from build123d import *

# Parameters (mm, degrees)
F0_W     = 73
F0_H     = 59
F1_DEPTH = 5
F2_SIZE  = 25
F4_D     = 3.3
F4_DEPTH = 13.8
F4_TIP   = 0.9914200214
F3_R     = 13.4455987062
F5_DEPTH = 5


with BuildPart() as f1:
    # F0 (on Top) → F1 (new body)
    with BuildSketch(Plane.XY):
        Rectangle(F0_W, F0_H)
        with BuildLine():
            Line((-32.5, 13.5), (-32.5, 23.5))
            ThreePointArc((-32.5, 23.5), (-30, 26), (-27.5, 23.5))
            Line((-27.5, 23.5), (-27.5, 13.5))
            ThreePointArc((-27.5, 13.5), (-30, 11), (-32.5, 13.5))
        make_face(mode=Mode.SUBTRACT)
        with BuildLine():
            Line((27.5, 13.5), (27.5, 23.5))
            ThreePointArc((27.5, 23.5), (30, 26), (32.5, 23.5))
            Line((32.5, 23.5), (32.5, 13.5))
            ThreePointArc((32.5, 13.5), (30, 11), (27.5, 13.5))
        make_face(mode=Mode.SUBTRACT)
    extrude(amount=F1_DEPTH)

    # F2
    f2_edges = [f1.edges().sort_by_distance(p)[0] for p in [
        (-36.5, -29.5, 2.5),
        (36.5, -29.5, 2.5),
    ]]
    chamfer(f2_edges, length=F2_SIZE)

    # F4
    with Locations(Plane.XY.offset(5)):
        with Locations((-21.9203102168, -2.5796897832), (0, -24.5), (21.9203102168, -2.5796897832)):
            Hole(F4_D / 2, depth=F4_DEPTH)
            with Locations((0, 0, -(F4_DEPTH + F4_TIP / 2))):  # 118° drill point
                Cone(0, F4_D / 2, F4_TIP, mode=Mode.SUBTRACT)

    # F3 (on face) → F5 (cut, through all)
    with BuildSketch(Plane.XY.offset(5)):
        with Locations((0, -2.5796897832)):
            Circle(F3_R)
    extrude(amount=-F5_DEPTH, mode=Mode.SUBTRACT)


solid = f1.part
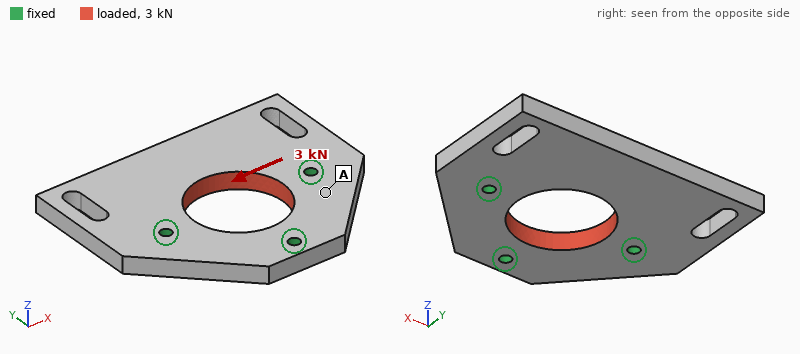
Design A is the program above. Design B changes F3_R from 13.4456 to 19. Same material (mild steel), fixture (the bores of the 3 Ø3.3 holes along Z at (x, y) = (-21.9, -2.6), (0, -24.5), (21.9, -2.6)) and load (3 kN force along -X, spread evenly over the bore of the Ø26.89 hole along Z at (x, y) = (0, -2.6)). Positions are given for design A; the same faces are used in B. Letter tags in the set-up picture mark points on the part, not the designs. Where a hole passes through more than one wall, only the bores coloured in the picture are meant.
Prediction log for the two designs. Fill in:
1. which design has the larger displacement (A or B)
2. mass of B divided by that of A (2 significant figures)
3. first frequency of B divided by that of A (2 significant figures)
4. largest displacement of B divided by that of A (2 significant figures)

B
0.81
0.88
2.5
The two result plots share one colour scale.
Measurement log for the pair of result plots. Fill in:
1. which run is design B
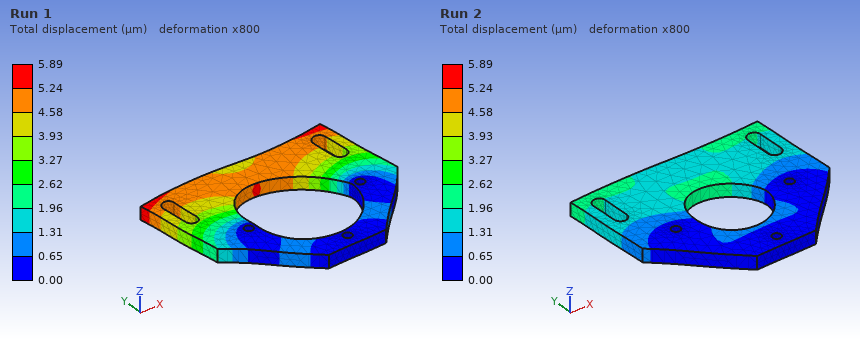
Run 1
